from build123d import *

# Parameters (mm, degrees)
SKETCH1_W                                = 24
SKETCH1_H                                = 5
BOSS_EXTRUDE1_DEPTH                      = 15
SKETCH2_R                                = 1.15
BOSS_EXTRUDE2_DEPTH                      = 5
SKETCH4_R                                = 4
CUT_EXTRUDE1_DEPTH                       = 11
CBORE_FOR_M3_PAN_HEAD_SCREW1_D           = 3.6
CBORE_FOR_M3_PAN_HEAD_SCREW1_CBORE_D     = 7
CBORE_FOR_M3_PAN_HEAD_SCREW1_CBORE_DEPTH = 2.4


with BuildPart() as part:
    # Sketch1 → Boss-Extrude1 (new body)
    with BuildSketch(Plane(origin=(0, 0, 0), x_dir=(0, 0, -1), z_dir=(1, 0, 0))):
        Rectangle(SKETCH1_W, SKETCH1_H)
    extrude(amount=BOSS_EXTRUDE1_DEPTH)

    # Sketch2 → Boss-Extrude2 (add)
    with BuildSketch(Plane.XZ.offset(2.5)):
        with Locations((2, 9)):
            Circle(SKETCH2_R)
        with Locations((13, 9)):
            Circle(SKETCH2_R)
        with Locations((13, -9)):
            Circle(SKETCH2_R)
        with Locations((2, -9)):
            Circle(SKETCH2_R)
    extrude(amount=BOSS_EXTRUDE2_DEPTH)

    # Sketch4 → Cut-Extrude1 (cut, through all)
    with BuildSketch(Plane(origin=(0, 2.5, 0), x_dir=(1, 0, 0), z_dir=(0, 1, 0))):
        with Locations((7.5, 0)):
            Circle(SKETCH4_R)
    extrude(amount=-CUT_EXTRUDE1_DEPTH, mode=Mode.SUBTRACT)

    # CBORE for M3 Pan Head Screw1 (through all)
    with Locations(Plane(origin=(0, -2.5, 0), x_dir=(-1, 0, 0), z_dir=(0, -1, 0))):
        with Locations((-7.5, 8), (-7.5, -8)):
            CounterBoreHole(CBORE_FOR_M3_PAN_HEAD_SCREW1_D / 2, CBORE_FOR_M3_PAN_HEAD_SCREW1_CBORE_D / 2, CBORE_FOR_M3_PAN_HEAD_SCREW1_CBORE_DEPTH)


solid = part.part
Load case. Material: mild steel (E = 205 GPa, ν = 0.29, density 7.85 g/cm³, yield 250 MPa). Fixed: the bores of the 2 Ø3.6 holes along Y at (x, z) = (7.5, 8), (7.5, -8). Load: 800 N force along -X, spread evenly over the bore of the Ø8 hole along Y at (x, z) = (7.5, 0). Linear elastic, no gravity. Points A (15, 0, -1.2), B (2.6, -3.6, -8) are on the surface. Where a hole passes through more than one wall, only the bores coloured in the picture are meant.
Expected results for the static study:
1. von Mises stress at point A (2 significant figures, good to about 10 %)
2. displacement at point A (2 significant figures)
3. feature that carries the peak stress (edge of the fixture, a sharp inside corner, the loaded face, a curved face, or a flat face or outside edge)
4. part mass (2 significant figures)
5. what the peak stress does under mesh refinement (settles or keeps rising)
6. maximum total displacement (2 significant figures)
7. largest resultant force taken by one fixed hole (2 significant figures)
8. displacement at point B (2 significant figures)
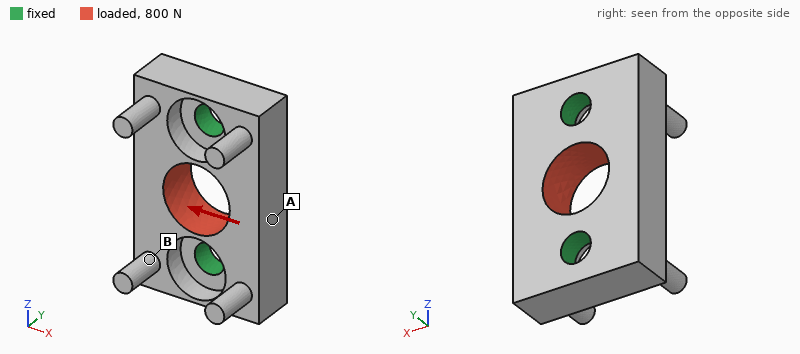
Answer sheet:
18 MPa
1.7 µm
edge of the fixture
11 g
keeps rising
2.1 µm
400 N
1.0 µm
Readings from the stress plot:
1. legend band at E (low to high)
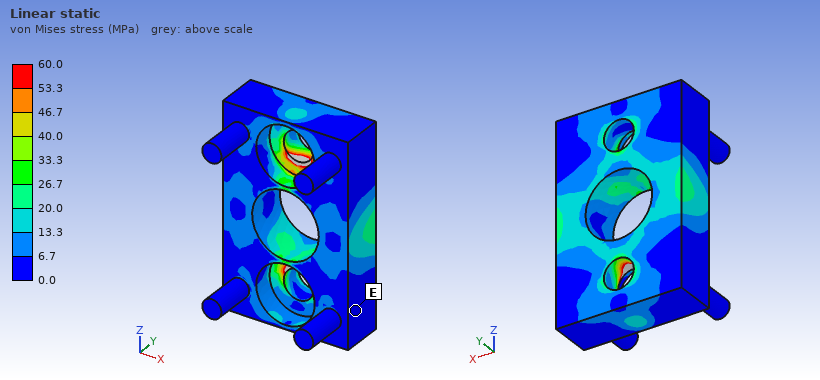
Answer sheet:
0.0 to 6.7 MPa
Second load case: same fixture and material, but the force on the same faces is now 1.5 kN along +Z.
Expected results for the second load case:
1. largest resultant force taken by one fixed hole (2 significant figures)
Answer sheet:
760 N
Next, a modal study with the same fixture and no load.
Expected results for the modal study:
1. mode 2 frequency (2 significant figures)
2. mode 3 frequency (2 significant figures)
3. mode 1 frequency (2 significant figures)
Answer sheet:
33 kHz
33 kHz
25 kHz
